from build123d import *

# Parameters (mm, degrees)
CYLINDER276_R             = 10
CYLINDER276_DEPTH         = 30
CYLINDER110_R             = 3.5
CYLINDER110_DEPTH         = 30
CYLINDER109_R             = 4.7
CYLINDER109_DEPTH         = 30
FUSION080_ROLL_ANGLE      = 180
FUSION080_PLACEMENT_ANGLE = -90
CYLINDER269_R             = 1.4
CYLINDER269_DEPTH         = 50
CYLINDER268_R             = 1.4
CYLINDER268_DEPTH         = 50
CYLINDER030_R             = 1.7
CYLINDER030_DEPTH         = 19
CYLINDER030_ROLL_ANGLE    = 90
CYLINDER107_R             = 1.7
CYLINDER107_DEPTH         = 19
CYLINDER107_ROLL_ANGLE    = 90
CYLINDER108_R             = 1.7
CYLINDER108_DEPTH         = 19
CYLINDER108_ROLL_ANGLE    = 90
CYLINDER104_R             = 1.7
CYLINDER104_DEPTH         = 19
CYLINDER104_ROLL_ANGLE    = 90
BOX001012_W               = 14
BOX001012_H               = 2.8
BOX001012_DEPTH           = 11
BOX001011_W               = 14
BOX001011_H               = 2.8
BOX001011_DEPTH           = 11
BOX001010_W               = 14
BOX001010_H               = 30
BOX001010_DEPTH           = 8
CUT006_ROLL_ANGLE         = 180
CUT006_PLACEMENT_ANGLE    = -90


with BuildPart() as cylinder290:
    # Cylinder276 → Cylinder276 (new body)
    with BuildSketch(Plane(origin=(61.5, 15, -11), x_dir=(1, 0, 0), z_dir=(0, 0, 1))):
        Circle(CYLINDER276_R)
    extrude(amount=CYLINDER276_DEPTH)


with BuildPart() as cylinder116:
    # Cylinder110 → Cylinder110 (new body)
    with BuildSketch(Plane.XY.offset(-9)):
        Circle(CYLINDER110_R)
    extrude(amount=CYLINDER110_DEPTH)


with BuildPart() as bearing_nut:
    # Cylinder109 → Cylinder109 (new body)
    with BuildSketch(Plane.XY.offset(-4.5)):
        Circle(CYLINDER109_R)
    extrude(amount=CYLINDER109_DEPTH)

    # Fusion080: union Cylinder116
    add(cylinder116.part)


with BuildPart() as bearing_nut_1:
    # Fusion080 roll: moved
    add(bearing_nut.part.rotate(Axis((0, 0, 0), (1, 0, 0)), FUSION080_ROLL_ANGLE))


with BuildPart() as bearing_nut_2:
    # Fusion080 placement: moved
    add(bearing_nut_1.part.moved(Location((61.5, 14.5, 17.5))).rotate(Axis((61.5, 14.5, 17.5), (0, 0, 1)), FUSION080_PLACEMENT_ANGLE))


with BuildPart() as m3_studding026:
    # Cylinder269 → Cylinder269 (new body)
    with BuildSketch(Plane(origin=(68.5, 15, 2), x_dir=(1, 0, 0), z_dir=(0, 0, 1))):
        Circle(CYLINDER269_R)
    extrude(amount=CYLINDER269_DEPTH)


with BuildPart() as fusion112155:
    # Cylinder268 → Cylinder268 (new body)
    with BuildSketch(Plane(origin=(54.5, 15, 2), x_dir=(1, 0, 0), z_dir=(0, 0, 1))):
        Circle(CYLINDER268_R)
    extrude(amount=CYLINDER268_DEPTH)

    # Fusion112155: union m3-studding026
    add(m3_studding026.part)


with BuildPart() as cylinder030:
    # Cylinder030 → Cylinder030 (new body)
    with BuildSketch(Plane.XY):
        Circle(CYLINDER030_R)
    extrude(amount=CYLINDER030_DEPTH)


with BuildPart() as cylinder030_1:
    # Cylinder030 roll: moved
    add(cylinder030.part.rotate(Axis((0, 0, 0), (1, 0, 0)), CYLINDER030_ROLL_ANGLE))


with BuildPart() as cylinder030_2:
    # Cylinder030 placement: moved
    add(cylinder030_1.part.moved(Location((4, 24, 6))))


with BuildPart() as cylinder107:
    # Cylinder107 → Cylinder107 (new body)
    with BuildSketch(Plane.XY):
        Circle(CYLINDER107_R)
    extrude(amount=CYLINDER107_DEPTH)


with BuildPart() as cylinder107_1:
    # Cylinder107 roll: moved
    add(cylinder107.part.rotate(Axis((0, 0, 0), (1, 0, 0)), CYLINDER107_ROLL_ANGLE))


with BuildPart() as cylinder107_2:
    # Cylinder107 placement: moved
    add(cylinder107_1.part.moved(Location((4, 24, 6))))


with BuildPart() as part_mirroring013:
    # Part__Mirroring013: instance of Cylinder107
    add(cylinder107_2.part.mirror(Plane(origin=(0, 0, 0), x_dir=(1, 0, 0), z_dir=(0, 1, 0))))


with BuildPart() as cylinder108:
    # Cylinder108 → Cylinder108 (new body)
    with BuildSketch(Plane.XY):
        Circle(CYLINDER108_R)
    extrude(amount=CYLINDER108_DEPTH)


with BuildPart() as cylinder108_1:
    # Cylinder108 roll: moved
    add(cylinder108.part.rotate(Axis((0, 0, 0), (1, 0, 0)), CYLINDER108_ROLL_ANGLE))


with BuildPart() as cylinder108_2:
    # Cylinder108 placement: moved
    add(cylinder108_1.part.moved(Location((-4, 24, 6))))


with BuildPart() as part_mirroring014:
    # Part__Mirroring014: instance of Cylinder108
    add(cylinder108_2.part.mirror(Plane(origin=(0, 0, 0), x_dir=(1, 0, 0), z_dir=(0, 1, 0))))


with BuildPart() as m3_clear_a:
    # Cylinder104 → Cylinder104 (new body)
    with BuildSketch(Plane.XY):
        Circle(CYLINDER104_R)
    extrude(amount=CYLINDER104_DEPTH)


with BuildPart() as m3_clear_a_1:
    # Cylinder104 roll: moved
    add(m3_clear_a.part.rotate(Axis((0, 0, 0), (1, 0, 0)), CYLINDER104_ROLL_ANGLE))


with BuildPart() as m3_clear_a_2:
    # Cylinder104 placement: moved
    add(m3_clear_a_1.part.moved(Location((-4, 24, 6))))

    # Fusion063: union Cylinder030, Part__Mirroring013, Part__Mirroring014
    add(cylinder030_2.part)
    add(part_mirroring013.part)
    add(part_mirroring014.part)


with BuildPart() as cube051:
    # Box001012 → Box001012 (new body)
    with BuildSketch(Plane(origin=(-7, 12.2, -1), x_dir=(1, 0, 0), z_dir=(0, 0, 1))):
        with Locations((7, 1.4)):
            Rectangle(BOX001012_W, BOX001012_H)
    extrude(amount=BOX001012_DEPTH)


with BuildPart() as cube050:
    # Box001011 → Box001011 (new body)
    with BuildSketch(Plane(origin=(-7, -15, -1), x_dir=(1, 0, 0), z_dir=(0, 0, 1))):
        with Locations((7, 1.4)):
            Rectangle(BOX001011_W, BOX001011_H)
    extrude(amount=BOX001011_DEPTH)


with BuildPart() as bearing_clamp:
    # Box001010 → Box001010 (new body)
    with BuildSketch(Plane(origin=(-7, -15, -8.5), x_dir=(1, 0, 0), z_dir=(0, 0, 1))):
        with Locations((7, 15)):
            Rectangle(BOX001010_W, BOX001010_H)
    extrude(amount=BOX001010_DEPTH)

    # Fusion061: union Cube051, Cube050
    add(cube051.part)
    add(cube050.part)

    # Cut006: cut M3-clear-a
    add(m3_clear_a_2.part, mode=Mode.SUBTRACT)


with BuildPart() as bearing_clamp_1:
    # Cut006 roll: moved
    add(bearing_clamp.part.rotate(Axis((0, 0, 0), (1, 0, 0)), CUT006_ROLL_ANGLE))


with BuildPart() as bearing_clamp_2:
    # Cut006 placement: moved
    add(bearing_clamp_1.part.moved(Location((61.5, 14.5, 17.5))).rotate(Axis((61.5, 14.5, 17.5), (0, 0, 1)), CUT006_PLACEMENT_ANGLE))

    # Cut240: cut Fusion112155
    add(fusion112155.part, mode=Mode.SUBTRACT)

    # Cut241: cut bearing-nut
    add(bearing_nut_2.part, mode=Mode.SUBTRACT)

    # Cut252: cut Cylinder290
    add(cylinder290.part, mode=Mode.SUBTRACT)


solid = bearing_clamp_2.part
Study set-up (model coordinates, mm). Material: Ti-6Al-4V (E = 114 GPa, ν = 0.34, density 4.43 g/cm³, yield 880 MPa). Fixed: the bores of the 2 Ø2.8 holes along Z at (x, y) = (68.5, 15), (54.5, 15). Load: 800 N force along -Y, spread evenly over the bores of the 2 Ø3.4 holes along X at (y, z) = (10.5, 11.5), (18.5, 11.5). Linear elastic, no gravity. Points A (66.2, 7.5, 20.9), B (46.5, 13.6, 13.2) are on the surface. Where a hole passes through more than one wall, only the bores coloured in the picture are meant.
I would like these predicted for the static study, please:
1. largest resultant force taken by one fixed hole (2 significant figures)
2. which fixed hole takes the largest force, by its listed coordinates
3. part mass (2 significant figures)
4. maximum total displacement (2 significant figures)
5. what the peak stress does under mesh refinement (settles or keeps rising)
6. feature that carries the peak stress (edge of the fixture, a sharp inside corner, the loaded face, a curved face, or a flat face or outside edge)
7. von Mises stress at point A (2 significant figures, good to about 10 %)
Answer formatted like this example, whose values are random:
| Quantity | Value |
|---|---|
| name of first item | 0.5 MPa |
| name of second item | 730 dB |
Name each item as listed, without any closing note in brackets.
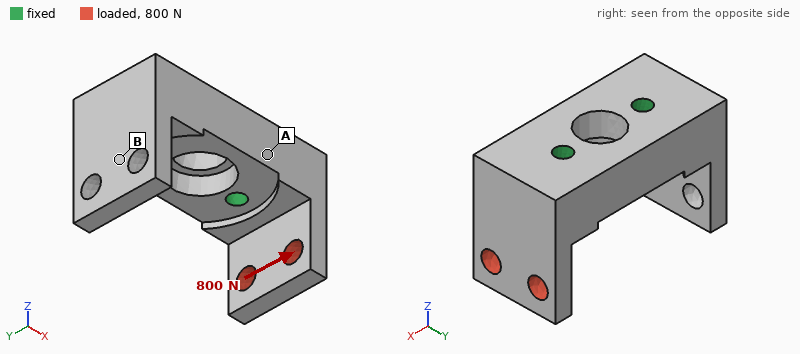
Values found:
| Quantity | Value |
|---|---|
| largest resultant force taken by one fixed hole | 980 N |
| which fixed hole takes the largest force, by its listed coordinates | (68.5, 15) |
| part mass | 15 g |
| maximum total displacement | 33 µm |
| what the peak stress does under mesh refinement | keeps rising |
| feature that carries the peak stress | edge of the fixture |
| von Mises stress at point A | 29 MPa |
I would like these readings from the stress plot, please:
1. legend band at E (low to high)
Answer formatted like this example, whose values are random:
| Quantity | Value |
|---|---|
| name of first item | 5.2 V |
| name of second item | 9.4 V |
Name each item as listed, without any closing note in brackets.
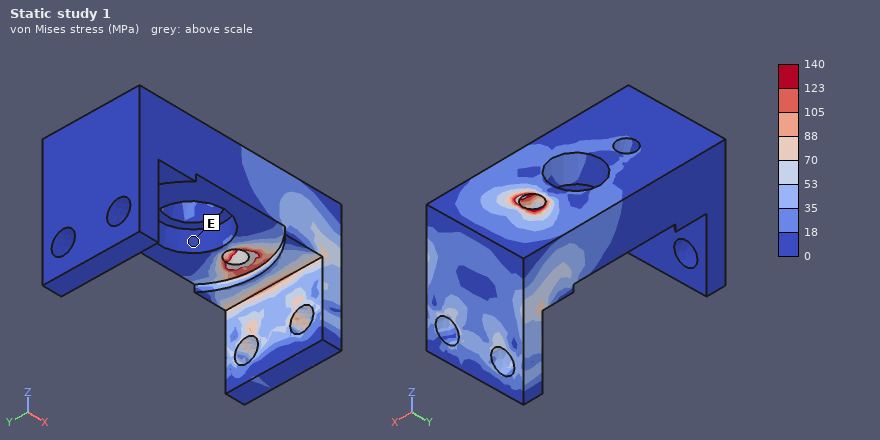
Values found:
| Quantity | Value |
|---|---|
| legend band at E | 0 to 18 MPa |
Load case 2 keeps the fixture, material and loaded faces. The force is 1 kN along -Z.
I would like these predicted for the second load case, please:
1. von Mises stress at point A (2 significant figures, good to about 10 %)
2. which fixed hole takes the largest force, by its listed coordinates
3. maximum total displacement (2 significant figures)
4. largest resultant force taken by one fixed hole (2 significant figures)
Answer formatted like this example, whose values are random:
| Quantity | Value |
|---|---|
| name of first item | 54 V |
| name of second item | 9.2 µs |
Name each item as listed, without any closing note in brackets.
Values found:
| Quantity | Value |
|---|---|
| von Mises stress at point A | 11 MPa |
| which fixed hole takes the largest force, by its listed coordinates | (68.5, 15) |
| maximum total displacement | 15 µm |
| largest resultant force taken by one fixed hole | 1.1 kN |
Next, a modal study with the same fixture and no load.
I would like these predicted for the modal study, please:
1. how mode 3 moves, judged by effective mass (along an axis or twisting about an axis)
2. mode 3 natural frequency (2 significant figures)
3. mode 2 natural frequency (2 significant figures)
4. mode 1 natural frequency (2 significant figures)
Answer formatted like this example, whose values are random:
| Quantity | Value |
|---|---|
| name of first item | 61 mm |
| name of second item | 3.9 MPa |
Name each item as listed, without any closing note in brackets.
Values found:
| Quantity | Value |
|---|---|
| how mode 3 moves, judged by effective mass | twisting about Z |
| mode 3 natural frequency | 23 kHz |
| mode 2 natural frequency | 15 kHz |
| mode 1 natural frequency | 15 kHz |
